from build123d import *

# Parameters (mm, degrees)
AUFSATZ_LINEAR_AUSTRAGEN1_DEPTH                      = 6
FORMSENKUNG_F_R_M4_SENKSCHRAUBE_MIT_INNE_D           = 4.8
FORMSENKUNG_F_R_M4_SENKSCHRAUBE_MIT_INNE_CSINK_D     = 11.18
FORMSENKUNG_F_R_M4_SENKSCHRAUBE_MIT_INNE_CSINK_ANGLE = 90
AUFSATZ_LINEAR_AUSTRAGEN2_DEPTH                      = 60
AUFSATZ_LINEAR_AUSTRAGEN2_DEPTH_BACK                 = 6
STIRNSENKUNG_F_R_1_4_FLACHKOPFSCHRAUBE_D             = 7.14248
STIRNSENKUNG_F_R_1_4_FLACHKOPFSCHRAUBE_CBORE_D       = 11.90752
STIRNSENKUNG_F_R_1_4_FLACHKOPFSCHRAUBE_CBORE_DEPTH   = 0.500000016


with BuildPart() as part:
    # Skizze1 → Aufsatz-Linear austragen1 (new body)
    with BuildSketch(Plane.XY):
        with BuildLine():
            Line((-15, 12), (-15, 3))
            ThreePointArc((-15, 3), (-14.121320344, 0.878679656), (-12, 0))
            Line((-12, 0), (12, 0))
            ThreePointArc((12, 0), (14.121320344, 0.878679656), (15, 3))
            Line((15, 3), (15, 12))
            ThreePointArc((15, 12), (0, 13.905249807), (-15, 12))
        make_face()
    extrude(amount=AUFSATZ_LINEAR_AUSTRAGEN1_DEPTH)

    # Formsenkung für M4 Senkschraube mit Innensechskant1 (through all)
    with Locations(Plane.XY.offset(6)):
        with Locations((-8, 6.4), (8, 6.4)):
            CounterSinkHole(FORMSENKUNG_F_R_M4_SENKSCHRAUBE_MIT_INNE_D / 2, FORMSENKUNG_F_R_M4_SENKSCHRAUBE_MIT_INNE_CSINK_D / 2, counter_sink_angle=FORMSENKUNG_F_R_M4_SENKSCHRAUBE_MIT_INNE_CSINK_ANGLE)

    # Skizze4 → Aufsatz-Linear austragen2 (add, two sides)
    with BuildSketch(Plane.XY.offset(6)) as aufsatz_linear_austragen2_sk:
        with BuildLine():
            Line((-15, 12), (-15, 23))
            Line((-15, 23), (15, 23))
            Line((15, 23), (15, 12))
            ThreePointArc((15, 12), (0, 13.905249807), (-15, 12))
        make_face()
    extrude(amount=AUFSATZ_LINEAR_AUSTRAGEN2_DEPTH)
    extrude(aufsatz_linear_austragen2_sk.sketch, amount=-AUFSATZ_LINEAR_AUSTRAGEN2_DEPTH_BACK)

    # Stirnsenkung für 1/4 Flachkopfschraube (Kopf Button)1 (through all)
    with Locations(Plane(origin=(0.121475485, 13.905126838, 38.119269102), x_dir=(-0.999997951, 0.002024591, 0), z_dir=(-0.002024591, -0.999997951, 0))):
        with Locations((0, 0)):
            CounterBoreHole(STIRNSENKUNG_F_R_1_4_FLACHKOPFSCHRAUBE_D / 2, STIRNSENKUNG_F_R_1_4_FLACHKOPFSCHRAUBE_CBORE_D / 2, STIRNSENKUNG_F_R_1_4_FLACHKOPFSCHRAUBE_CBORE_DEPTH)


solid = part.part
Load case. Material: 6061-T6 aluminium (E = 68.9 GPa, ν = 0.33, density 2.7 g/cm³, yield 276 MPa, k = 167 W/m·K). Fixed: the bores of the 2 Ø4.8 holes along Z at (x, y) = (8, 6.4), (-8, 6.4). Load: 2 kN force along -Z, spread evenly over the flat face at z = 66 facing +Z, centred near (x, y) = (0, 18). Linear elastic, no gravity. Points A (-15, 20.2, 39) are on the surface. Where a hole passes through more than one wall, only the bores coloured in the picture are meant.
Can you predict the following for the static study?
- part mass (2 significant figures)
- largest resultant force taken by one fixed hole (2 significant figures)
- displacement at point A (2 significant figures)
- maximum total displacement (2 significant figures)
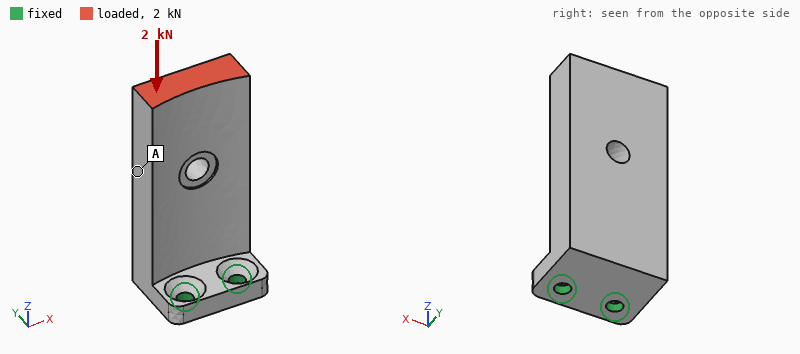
56 g
1.0 kN
0.26 mm
0.44 mm
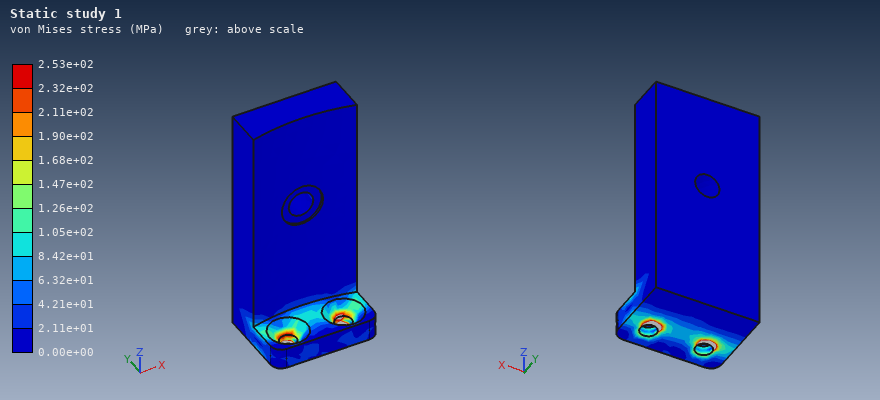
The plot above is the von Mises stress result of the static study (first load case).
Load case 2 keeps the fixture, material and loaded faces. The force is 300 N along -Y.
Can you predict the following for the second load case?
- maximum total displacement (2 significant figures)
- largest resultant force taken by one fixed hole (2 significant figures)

0.65 mm
150 N
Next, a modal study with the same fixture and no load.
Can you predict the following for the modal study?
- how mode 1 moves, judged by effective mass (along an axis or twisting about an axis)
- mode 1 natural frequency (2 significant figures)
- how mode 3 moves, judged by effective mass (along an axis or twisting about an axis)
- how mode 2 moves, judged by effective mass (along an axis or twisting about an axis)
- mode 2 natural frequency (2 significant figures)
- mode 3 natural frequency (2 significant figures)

along Y
870 Hz
along Z
along X
2100 Hz
6200 Hz
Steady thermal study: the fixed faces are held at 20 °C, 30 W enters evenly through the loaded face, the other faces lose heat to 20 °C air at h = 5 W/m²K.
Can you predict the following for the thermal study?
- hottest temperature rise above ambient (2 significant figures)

50 K
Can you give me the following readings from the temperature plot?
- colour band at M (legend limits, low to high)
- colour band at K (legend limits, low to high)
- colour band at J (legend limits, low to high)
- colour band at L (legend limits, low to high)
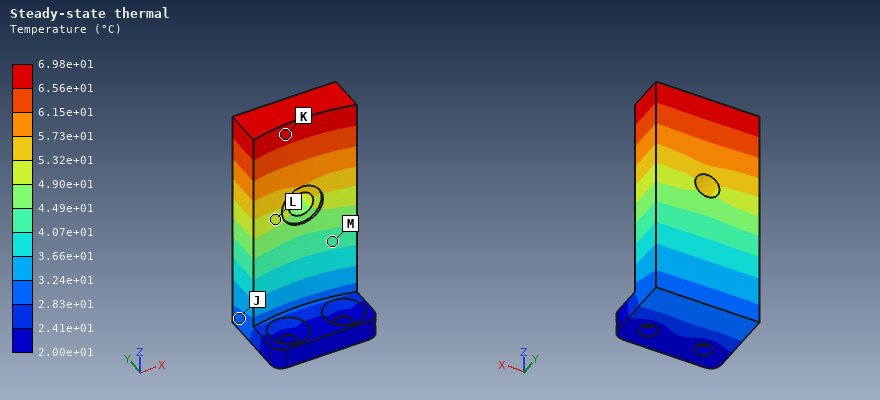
4.07e+01 to 4.49e+01 °C
6.56e+01 to 6.98e+01 °C
2.83e+01 to 3.24e+01 °C
4.90e+01 to 5.32e+01 °C
